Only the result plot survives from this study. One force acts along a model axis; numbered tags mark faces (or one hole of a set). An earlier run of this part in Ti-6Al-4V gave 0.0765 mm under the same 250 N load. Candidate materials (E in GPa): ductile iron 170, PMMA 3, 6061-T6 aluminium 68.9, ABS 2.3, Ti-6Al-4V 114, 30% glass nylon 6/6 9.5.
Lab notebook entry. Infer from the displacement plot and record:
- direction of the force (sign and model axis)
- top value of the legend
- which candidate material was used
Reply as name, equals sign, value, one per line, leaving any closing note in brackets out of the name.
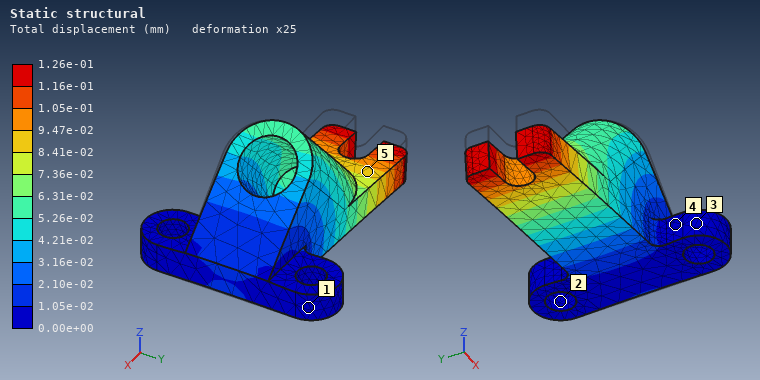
direction of the force = -Z
top value of the legend = 1.26e-01 mm
which candidate material was used = 6061-T6 aluminium
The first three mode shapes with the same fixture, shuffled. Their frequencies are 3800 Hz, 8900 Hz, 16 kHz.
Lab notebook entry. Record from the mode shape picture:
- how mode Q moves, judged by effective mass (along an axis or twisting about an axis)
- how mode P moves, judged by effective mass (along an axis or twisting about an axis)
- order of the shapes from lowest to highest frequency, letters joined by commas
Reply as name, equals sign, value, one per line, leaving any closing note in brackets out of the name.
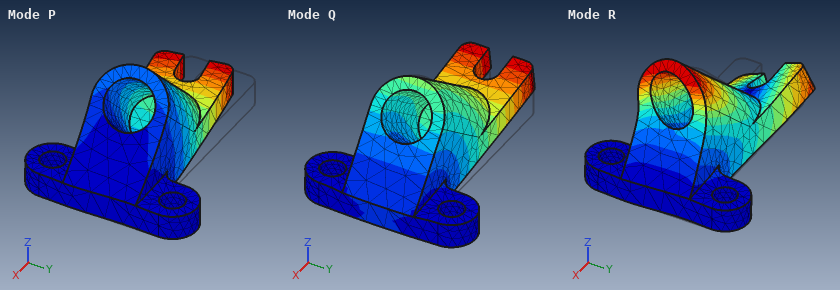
how mode Q moves, judged by effective mass = along Z
how mode P moves, judged by effective mass = along Y
order of the shapes from lowest to highest frequency, letters joined by commas = Q, P, R
